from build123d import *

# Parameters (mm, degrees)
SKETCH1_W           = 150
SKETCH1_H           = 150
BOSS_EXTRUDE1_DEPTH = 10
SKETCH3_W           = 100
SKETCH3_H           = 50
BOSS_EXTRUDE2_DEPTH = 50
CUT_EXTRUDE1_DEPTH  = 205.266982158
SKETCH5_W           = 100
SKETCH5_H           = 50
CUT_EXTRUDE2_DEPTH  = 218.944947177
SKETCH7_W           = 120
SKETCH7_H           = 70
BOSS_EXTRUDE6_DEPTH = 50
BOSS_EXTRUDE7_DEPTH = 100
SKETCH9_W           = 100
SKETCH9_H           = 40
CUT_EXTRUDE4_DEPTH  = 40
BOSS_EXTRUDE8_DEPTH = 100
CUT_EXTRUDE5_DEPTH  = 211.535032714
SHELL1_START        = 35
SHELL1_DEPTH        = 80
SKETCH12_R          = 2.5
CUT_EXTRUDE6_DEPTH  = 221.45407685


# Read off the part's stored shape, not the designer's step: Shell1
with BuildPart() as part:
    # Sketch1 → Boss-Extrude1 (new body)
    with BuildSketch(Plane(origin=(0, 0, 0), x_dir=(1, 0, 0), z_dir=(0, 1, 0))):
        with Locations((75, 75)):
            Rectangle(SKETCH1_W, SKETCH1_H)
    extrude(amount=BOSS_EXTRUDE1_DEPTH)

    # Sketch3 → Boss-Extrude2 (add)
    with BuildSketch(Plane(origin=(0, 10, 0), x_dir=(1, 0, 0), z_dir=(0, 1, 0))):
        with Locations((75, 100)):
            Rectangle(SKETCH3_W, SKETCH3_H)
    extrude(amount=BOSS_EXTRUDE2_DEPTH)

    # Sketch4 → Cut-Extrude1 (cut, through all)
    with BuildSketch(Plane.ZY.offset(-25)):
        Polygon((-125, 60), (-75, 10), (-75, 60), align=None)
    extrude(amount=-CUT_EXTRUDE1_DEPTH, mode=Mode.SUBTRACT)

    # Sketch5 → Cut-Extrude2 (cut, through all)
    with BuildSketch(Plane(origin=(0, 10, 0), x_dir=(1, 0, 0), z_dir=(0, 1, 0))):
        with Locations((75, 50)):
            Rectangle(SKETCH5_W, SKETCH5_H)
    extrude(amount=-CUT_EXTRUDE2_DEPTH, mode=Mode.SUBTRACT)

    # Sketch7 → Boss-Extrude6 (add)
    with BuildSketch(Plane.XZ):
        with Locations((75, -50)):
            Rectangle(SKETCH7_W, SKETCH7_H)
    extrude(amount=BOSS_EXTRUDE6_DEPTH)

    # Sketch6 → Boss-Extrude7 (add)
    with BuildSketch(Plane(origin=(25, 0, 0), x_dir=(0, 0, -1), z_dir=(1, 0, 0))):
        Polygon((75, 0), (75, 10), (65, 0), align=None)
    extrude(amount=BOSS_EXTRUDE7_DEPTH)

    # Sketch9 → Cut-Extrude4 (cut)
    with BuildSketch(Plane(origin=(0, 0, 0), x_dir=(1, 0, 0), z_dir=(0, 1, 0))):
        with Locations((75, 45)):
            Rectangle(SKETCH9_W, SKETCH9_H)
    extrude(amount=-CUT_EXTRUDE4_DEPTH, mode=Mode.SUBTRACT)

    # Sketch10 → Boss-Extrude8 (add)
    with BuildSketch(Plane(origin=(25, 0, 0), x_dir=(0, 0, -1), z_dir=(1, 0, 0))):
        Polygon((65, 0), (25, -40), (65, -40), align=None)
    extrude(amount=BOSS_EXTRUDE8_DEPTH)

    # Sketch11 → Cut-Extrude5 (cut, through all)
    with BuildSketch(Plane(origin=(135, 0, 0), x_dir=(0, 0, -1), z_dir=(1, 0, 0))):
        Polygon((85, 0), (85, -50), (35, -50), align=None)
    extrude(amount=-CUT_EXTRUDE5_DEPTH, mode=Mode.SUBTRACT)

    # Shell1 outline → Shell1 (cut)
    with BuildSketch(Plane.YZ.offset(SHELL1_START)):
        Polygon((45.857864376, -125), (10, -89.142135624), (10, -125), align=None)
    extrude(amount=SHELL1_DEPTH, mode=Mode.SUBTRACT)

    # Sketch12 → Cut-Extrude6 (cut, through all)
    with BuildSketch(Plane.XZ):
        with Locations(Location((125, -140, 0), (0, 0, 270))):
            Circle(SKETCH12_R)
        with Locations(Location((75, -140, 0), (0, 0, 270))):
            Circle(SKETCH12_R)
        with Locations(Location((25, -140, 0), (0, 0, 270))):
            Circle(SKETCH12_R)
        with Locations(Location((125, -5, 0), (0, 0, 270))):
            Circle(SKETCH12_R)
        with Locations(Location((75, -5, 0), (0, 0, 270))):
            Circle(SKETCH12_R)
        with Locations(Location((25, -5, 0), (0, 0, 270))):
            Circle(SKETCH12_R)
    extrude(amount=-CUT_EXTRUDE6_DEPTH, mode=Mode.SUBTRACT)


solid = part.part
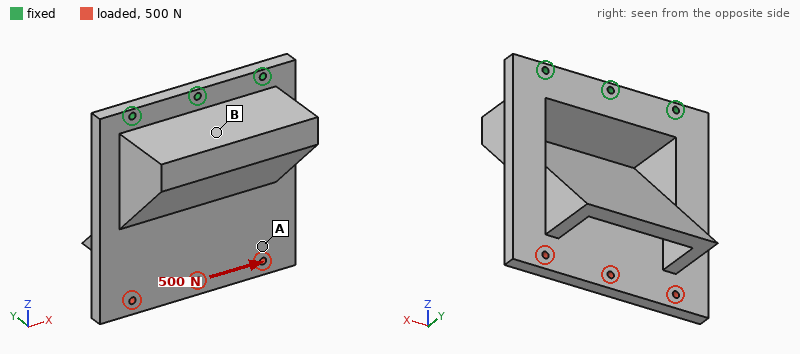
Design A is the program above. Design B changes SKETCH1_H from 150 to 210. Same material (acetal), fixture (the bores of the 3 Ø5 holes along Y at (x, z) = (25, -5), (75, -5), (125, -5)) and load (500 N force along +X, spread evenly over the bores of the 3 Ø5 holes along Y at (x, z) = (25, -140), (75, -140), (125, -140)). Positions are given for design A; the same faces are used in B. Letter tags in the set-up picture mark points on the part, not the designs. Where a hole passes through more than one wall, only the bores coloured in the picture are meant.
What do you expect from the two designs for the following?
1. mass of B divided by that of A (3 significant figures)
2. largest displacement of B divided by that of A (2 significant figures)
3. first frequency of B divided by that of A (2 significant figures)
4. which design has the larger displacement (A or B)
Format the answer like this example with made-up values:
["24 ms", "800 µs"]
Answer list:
["1.20", "0.77", "0.89", "A"]
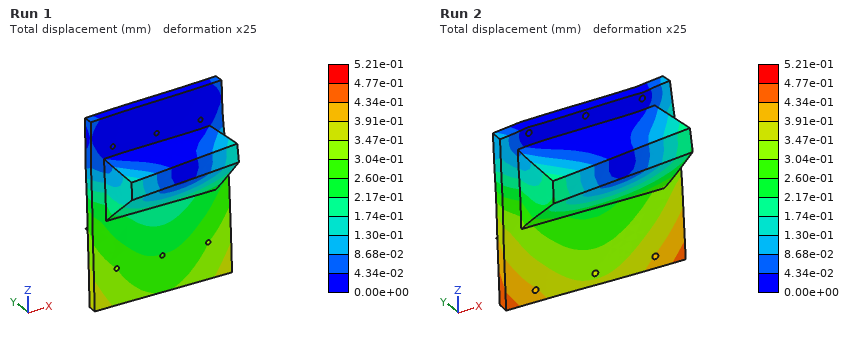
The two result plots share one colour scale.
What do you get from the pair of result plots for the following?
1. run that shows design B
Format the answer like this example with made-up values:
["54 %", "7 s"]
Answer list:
["Run 1"]
